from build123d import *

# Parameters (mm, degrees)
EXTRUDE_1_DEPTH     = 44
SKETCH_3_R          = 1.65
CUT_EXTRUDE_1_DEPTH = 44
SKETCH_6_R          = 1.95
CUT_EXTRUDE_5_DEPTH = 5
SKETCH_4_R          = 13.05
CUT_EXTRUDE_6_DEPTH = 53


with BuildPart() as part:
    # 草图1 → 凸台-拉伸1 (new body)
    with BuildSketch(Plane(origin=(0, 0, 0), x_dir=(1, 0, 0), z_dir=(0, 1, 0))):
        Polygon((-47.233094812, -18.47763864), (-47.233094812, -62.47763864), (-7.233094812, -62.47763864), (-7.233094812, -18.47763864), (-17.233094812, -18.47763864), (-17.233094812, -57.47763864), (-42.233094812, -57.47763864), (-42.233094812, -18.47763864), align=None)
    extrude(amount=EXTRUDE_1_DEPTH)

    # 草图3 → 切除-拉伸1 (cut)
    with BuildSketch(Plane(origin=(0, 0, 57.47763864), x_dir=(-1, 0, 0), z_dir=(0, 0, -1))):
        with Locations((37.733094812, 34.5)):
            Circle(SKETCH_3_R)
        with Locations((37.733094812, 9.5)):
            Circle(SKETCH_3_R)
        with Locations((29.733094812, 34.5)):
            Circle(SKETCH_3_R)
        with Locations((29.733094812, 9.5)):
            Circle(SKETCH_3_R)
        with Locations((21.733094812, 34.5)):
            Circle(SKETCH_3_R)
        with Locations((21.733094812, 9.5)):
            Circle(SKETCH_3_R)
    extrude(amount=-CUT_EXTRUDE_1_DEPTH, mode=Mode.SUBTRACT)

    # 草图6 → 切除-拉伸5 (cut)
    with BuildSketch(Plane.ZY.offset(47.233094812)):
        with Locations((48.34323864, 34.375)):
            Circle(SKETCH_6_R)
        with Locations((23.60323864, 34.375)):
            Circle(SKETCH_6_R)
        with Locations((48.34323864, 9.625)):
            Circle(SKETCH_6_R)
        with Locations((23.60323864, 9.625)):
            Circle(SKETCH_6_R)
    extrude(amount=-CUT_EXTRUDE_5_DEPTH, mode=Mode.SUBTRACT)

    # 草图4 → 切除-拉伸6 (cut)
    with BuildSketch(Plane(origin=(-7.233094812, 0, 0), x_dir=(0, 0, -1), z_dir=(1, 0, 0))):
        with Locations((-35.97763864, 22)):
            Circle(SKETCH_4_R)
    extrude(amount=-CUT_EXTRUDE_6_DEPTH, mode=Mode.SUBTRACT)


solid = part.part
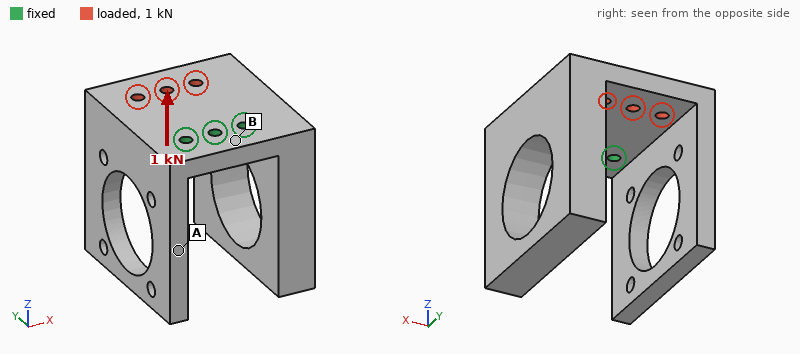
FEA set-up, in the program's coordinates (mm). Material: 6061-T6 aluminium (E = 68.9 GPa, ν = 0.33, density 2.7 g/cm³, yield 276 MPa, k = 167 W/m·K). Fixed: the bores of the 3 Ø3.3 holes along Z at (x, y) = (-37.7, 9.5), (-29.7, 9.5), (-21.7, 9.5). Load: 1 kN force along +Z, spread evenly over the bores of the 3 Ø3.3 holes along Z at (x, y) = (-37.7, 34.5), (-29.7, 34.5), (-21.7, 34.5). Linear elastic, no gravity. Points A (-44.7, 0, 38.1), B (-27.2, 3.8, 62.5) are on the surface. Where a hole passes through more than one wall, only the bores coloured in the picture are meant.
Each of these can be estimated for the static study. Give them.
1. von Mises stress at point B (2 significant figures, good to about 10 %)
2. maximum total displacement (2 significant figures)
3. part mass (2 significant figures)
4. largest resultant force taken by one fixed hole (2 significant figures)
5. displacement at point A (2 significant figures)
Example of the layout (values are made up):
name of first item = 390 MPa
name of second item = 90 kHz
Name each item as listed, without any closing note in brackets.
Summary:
von Mises stress at point B = 30 MPa
maximum total displacement = 0.19 mm
part mass = 70 g
largest resultant force taken by one fixed hole = 370 N
displacement at point A = 0.075 mm
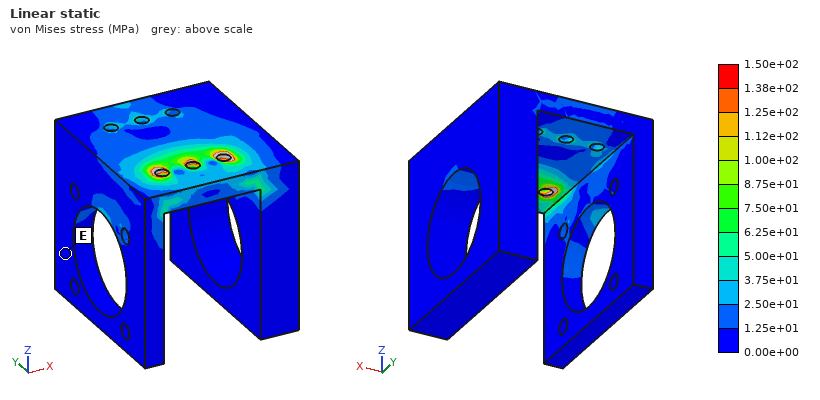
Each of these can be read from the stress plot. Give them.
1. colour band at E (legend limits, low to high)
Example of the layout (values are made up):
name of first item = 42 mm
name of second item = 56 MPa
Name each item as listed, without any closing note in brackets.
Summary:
colour band at E = 0.00e+00 to 1.25e+01 MPa
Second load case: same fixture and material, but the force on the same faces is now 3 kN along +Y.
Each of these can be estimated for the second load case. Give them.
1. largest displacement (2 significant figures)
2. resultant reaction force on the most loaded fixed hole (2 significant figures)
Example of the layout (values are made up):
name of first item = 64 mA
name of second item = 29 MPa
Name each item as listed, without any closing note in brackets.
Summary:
largest displacement = 9.5 µm
resultant reaction force on the most loaded fixed hole = 1.2 kN
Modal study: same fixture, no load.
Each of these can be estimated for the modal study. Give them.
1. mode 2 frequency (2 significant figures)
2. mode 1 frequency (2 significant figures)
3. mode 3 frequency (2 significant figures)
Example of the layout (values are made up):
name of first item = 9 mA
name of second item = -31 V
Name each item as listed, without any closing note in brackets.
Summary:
mode 2 frequency = 1800 Hz
mode 1 frequency = 1500 Hz
mode 3 frequency = 1900 Hz
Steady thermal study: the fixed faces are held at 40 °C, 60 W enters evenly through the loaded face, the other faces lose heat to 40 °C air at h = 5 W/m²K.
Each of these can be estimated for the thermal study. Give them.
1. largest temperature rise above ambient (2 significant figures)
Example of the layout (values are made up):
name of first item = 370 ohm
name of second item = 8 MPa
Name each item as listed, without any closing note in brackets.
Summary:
largest temperature rise above ambient = 44 K
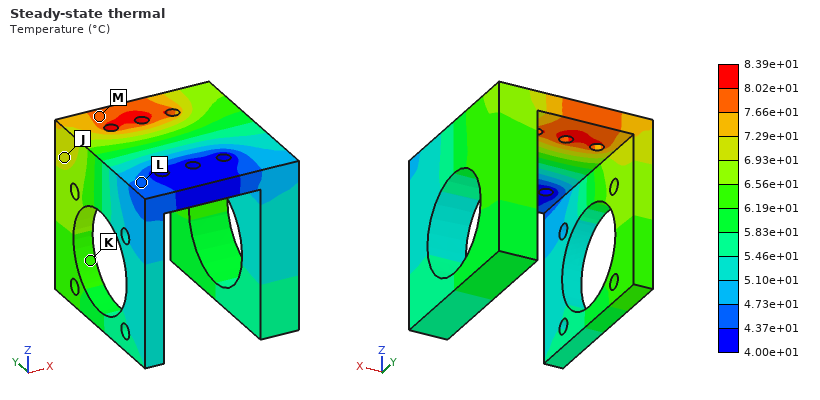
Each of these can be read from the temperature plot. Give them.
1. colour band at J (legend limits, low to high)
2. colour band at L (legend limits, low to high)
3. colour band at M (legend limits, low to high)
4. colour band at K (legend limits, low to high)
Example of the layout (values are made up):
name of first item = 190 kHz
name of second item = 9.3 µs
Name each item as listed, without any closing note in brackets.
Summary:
colour band at J = 6.93e+01 to 7.29e+01 °C
colour band at L = 4.37e+01 to 4.73e+01 °C
colour band at M = 7.66e+01 to 8.02e+01 °C
colour band at K = 6.19e+01 to 6.56e+01 °C
